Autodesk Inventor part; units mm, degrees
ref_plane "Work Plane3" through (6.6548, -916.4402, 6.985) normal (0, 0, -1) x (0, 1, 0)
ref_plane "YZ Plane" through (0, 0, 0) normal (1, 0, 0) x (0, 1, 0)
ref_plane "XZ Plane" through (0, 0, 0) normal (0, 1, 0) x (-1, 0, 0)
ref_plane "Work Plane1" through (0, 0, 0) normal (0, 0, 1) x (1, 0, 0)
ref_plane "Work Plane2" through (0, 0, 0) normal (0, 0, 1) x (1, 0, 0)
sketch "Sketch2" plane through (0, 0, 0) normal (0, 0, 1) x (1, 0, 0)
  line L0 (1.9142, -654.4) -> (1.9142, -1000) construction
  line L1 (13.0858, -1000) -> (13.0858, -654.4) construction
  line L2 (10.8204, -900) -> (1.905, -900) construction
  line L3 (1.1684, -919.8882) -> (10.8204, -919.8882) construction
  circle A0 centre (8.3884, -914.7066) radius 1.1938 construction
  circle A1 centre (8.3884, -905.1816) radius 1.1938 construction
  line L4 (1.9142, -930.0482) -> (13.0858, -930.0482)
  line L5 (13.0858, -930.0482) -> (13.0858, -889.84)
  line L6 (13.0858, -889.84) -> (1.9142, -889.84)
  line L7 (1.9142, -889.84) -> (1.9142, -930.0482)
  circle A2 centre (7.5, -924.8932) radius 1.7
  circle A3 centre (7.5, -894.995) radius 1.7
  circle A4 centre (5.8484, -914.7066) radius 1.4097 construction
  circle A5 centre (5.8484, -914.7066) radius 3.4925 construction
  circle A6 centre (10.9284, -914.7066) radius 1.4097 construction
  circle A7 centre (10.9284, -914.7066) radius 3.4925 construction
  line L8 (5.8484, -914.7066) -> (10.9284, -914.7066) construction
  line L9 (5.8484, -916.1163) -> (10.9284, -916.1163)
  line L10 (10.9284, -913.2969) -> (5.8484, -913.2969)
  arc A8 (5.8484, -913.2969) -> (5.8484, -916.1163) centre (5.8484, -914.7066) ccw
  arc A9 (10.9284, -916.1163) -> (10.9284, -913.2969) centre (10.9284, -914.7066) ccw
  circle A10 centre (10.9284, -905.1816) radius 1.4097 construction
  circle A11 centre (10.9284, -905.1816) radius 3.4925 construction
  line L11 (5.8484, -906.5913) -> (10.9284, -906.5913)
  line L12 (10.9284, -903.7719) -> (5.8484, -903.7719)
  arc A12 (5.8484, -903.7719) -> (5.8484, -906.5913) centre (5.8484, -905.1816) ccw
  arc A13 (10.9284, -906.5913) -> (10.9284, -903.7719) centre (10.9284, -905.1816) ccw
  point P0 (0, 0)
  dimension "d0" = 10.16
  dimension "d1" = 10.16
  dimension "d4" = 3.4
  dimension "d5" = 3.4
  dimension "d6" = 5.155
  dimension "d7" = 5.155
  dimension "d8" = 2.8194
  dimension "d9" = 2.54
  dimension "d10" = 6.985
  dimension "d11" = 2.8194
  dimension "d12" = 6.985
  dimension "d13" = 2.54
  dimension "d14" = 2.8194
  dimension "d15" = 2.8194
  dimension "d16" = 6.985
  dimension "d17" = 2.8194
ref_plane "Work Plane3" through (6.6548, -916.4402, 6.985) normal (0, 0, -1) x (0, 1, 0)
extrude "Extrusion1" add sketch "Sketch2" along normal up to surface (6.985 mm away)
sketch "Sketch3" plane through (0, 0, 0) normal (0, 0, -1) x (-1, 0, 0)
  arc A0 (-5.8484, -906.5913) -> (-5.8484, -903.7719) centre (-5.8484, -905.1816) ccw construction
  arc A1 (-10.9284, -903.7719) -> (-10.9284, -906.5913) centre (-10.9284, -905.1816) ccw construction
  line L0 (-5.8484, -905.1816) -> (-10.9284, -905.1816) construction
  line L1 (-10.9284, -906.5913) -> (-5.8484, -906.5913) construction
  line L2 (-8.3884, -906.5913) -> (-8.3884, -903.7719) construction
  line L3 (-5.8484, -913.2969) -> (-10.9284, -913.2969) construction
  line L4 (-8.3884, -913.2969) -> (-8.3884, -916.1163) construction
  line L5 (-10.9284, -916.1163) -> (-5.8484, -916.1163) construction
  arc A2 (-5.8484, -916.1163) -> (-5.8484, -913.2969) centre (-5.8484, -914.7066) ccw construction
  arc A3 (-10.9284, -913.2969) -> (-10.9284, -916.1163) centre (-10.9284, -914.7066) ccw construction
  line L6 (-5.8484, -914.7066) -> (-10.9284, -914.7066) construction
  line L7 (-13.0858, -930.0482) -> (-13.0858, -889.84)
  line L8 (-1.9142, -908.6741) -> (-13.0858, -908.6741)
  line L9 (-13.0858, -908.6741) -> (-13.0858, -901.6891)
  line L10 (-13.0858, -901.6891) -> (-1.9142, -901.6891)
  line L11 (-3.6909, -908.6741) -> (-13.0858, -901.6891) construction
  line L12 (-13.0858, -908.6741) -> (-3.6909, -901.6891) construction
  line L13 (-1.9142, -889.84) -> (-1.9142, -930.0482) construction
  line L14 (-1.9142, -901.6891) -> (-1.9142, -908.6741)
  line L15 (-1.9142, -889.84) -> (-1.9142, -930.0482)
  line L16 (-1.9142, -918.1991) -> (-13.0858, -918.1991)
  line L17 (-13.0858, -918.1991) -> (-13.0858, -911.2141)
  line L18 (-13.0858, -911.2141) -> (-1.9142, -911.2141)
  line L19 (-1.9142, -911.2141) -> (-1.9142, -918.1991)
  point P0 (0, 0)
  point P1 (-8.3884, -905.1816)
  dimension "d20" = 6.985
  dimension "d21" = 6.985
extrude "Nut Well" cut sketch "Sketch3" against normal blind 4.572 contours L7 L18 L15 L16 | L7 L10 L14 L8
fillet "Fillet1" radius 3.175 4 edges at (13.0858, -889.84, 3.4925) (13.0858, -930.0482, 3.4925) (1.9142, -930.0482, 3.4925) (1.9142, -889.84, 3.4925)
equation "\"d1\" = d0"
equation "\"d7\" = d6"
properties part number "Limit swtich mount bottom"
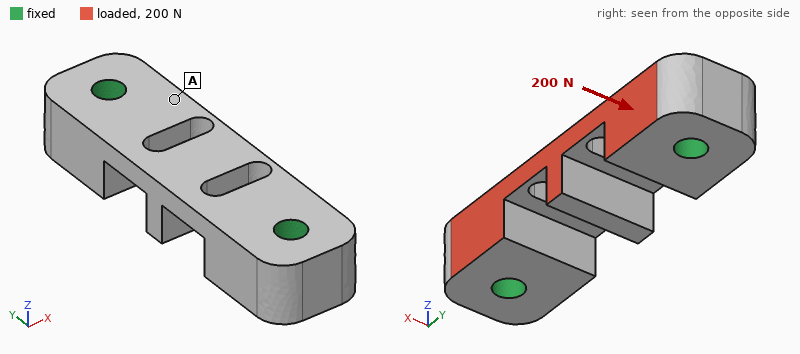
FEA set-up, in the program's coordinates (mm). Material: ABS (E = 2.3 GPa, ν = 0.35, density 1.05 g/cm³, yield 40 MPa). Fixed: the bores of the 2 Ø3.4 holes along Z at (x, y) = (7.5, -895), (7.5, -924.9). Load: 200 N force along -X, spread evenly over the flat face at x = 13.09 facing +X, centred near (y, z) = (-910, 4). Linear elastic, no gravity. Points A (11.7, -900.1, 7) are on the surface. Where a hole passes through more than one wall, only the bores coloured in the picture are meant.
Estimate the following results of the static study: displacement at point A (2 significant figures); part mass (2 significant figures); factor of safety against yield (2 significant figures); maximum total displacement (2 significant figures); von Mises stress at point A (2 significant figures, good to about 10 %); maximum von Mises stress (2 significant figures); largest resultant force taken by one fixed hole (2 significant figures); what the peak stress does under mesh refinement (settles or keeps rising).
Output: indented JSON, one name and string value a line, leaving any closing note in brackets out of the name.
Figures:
{
  "displacement at point A": "17 µm",
  "part mass": "2.2 g",
  "factor of safety against yield": "2.1",
  "maximum total displacement": "90 µm",
  "von Mises stress at point A": "1.7 MPa",
  "maximum von Mises stress": "19 MPa",
  "largest resultant force taken by one fixed hole": "100 N",
  "what the peak stress does under mesh refinement": "settles"
}
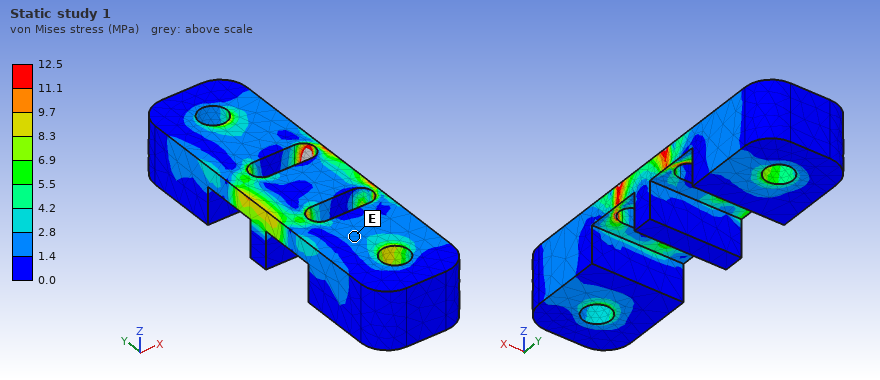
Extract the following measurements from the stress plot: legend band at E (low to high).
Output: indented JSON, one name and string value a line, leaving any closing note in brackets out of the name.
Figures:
{
  "legend band at E": "1.4 to 2.8 MPa"
}
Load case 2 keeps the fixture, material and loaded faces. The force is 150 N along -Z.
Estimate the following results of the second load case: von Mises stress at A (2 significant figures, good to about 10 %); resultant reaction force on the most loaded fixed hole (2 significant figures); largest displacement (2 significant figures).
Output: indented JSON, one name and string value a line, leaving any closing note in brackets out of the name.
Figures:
{
  "von Mises stress at A": "8.5 MPa",
  "resultant reaction force on the most loaded fixed hole": "75 N",
  "largest displacement": "0.23 mm"
}
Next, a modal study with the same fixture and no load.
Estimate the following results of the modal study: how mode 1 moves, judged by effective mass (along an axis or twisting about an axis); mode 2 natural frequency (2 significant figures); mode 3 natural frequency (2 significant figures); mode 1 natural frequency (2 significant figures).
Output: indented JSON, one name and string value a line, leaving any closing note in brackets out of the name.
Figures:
{
  "how mode 1 moves, judged by effective mass": "along Z",
  "mode 2 natural frequency": "6500 Hz",
  "mode 3 natural frequency": "8900 Hz",
  "mode 1 natural frequency": "5700 Hz"
}
